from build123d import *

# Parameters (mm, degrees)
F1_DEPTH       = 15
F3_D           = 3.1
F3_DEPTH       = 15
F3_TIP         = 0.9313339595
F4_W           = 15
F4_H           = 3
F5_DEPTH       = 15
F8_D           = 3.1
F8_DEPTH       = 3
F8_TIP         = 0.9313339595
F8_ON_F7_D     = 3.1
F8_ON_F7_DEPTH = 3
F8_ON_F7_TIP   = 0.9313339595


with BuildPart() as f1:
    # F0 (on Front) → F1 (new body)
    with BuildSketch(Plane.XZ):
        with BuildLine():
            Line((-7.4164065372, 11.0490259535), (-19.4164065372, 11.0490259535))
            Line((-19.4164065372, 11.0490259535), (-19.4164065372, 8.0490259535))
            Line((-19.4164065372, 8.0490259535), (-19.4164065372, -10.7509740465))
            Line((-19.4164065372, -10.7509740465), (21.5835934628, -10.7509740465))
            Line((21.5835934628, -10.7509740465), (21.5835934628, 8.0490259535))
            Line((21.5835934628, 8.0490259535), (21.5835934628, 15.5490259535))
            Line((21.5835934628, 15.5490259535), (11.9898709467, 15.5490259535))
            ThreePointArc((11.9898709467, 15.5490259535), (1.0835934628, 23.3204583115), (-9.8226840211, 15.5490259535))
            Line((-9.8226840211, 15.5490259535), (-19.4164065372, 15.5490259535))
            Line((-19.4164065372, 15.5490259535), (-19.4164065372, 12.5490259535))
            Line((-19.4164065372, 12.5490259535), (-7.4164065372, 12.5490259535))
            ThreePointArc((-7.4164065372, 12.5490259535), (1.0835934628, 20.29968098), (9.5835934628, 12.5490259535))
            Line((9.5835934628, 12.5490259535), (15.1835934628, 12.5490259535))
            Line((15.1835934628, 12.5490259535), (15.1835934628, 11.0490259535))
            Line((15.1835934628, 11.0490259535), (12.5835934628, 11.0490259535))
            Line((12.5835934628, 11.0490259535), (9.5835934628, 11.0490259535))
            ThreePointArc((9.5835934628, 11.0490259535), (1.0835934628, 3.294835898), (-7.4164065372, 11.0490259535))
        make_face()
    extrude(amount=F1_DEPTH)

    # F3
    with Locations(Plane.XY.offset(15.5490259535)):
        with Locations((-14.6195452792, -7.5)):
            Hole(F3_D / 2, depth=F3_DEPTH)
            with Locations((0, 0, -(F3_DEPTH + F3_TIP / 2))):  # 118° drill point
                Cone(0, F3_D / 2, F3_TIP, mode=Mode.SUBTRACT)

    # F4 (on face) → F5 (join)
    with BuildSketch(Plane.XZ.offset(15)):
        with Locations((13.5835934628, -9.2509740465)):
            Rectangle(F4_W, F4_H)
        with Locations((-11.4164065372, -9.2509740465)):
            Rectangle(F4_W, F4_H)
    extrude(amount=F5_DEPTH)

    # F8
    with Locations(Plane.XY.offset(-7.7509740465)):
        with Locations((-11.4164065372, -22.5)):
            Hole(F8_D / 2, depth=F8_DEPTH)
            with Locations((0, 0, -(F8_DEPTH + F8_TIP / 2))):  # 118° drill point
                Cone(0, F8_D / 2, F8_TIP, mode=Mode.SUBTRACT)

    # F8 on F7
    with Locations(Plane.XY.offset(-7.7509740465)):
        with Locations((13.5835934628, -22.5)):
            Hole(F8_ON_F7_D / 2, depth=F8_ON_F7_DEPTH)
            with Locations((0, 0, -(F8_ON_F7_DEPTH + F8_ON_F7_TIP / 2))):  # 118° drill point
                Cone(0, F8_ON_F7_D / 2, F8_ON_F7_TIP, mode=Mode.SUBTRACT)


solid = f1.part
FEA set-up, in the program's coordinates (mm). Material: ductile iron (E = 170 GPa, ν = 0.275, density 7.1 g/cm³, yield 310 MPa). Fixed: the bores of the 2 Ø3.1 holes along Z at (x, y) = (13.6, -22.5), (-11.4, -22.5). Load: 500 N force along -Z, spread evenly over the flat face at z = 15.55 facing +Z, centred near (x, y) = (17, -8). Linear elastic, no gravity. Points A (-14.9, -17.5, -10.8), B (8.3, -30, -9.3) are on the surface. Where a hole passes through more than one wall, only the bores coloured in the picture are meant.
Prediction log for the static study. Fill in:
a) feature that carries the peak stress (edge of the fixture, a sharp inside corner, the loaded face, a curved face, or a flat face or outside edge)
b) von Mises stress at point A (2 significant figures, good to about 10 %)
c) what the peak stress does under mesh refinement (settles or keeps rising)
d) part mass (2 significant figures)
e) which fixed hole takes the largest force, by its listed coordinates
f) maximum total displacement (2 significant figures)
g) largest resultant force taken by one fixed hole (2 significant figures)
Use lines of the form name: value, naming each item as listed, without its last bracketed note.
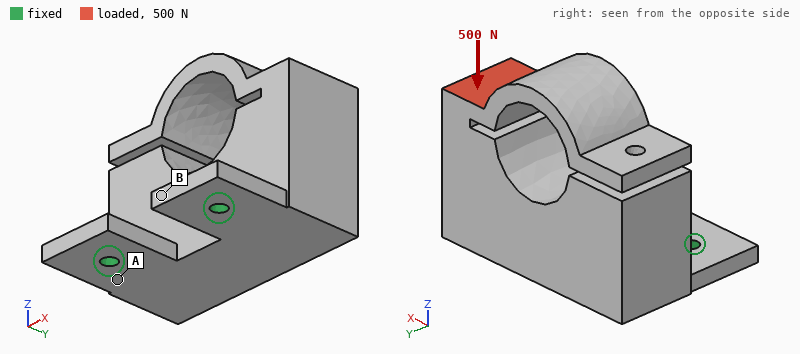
feature that carries the peak stress: edge of the fixture
von Mises stress at point A: 100 MPa
what the peak stress does under mesh refinement: keeps rising
part mass: 110 g
which fixed hole takes the largest force, by its listed coordinates: (13.6, -22.5)
maximum total displacement: 0.16 mm
largest resultant force taken by one fixed hole: 530 N
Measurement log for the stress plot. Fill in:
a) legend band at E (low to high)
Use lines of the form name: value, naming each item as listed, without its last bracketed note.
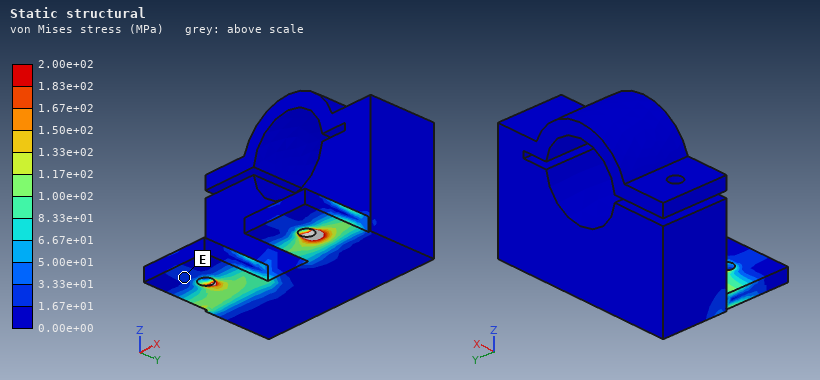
legend band at E: 1.67e+01 to 3.33e+01 MPa
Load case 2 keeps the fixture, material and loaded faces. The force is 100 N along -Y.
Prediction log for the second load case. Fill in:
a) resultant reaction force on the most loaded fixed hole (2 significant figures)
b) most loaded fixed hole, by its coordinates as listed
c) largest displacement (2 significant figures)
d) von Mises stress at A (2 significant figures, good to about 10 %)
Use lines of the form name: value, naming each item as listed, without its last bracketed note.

resultant reaction force on the most loaded fixed hole: 110 N
most loaded fixed hole, by its coordinates as listed: (13.6, -22.5)
largest displacement: 72 µm
von Mises stress at A: 48 MPa
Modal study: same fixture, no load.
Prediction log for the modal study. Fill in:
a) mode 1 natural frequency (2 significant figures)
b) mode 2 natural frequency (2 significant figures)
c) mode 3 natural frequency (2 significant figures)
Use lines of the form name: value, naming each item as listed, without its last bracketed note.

mode 1 natural frequency: 980 Hz
mode 2 natural frequency: 1600 Hz
mode 3 natural frequency: 3200 Hz
